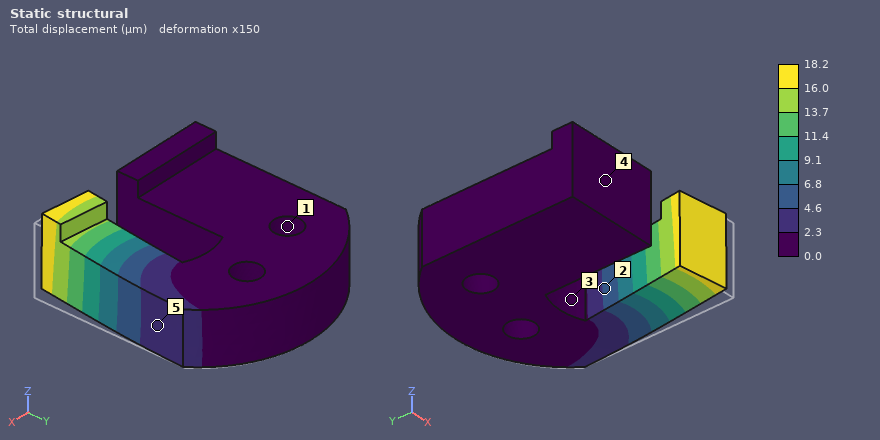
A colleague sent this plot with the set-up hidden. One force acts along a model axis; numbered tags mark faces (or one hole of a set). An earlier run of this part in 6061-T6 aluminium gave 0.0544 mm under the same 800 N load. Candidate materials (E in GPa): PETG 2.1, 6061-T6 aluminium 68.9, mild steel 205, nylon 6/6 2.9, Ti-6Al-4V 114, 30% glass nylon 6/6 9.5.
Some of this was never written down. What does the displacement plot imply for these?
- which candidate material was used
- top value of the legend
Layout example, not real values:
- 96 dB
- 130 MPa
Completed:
- mild steel
- 18.2 µm
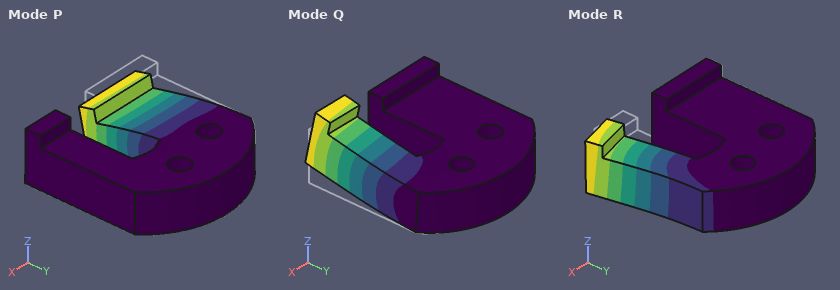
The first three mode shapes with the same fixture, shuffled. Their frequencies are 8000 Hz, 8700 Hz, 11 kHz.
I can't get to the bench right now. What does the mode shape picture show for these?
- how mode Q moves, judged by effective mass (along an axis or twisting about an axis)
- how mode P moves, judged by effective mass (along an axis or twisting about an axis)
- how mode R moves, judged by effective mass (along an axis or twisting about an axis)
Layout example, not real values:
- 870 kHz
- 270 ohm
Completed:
- along Z
- along Z
- along X
